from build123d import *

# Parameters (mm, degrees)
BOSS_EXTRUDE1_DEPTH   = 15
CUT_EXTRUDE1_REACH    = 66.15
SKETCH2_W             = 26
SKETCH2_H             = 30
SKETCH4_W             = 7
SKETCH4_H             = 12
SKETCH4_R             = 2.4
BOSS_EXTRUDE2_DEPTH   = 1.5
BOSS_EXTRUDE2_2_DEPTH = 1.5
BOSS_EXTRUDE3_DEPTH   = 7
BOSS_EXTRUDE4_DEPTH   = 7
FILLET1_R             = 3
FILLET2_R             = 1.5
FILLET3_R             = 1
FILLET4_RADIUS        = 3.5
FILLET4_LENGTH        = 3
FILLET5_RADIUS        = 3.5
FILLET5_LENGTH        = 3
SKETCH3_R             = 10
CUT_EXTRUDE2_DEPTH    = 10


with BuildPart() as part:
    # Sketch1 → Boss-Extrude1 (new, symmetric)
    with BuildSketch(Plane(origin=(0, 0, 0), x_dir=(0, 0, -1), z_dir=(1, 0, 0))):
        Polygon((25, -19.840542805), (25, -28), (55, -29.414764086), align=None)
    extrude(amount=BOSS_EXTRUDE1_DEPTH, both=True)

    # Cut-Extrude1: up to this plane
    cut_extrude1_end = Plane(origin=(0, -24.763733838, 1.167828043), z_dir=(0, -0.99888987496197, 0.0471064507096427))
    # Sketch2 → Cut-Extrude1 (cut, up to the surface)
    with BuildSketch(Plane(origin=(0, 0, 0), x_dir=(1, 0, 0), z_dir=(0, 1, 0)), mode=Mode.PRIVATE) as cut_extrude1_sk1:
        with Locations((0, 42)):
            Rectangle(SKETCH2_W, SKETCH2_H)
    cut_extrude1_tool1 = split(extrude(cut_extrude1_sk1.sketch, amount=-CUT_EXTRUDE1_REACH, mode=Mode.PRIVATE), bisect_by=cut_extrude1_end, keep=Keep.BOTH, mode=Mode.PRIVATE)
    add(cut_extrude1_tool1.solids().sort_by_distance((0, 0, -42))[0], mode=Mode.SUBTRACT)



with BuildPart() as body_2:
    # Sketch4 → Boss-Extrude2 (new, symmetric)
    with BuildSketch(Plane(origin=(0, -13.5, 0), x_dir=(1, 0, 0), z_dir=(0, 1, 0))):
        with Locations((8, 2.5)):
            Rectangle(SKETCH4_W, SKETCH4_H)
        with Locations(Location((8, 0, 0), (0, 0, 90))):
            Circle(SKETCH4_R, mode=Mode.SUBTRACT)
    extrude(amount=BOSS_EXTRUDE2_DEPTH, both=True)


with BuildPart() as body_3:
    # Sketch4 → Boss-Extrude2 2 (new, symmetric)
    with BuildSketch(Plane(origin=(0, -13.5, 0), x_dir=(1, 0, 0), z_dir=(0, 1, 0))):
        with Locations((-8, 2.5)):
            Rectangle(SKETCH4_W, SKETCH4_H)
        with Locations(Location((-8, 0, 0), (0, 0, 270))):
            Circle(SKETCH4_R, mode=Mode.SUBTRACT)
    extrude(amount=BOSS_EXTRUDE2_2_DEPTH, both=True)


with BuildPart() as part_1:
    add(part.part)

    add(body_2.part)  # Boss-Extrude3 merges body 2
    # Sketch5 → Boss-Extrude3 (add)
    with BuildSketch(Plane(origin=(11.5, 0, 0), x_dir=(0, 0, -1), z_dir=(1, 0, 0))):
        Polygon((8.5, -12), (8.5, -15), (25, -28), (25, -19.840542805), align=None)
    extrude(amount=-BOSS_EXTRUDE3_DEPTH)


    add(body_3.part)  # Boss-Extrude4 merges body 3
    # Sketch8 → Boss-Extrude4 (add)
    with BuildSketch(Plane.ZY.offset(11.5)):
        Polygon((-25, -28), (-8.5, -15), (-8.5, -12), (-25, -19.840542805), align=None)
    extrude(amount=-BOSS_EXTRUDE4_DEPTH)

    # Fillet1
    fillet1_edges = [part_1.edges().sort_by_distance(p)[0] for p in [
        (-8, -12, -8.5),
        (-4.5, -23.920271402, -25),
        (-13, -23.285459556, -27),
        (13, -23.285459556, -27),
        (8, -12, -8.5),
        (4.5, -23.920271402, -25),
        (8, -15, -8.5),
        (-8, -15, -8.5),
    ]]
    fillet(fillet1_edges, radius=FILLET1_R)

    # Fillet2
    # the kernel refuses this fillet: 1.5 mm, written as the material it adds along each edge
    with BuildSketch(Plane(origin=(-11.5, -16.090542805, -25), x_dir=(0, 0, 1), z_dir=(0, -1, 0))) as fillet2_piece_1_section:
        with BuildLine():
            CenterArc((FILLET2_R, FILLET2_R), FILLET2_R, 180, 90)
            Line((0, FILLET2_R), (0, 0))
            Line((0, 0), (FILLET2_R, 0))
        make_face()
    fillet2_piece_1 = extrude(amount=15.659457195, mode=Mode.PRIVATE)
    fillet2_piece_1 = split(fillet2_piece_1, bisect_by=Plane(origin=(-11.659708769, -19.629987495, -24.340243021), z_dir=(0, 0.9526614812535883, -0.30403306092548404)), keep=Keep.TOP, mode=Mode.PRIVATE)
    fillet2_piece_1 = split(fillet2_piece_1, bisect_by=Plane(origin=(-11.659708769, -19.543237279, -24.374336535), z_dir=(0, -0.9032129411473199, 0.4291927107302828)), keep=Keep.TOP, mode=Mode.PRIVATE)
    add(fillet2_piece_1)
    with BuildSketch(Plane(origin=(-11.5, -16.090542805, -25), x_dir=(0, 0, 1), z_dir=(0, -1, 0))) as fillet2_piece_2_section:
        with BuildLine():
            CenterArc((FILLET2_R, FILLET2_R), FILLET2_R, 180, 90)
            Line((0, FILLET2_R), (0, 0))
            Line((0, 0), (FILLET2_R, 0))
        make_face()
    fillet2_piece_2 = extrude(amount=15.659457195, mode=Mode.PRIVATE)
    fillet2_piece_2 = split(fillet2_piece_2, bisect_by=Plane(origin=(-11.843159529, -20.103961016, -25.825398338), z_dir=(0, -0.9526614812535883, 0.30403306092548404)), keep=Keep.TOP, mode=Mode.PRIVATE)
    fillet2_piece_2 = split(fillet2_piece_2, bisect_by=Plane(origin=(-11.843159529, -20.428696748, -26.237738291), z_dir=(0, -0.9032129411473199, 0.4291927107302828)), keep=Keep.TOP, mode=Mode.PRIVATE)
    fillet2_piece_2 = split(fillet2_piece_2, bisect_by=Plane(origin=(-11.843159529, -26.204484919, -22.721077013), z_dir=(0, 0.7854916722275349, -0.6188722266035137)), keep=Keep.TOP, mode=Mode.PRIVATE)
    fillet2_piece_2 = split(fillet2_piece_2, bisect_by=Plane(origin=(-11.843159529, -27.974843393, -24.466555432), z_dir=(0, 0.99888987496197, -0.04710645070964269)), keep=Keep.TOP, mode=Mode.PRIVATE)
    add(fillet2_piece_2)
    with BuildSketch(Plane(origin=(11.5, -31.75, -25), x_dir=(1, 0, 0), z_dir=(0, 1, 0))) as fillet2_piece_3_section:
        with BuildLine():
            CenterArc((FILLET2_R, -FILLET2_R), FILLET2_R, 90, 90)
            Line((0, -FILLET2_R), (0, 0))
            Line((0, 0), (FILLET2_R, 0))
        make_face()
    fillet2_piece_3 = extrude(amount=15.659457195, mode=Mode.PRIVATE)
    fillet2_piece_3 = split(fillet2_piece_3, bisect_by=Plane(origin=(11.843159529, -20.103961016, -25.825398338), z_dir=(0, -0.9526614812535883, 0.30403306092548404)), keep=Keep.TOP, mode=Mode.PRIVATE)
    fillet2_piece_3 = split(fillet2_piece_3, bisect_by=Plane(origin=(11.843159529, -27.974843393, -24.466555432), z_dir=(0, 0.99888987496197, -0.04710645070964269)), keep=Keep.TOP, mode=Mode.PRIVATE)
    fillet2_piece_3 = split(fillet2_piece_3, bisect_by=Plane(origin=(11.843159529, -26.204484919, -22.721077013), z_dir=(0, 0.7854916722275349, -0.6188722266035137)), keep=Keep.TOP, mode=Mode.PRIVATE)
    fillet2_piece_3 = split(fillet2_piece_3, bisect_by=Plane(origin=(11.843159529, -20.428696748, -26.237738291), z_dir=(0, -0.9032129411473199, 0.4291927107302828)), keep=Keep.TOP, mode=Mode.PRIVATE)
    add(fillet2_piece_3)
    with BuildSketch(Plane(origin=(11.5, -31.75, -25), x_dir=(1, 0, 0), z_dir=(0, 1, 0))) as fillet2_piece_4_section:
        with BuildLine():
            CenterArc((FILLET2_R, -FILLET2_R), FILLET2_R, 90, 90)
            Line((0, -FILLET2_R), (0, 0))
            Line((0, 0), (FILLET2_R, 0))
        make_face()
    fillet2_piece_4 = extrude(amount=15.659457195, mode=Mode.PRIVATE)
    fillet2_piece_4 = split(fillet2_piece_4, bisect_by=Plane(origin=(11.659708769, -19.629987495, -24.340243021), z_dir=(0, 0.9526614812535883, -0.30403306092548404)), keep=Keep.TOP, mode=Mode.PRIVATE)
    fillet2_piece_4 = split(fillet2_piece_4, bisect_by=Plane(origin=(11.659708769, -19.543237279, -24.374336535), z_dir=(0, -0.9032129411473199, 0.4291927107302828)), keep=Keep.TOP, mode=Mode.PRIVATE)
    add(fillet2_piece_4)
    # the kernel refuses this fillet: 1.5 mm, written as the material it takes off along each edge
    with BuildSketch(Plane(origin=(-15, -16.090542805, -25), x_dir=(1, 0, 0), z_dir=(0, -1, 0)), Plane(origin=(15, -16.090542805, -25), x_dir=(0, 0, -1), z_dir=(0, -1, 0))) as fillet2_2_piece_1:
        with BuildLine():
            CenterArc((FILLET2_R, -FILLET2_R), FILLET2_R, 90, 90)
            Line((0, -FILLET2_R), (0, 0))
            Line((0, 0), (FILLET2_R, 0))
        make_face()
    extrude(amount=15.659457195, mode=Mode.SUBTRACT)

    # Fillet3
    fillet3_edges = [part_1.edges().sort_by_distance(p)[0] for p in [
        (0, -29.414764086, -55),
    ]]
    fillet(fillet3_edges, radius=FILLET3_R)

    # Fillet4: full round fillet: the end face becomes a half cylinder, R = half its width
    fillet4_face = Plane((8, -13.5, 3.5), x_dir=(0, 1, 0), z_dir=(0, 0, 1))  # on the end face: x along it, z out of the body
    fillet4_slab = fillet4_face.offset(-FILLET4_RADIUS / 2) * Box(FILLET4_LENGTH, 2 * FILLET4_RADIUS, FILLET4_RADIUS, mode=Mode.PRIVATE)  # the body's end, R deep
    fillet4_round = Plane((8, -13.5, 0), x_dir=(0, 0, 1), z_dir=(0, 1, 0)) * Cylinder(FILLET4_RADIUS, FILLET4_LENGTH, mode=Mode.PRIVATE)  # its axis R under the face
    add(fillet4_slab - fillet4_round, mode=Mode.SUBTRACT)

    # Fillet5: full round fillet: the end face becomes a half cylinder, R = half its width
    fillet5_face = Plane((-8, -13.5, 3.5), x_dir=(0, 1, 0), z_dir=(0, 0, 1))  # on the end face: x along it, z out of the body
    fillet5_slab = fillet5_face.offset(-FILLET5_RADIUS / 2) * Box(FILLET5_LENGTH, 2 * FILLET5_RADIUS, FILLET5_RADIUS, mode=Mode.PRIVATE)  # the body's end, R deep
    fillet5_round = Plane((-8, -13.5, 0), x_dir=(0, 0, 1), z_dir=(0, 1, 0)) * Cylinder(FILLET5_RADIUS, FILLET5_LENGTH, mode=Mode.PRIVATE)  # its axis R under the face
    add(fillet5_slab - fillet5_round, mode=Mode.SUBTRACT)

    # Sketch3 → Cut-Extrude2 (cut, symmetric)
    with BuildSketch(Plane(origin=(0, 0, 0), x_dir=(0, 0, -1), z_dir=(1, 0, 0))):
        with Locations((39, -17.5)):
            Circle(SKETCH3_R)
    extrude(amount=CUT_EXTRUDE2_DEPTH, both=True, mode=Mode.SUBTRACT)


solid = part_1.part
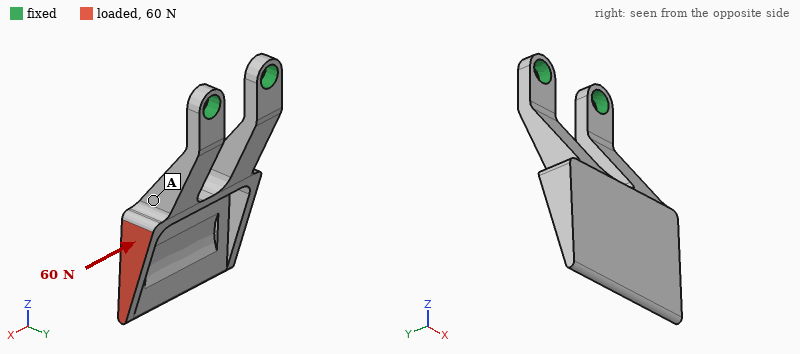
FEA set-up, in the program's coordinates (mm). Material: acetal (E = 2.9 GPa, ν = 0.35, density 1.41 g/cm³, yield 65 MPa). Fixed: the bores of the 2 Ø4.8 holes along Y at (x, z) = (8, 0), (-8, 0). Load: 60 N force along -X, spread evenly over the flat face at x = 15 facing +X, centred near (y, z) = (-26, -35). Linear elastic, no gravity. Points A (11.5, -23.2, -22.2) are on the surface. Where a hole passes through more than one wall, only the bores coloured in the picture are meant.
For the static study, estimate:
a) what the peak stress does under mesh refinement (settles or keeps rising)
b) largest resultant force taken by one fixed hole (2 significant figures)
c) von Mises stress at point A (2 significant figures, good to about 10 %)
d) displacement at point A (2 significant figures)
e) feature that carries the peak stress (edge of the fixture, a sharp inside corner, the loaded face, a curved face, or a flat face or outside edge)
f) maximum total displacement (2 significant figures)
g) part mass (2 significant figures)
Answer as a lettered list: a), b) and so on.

a) keeps rising
b) 87 N
c) 3.0 MPa
d) 0.31 mm
e) edge of the fixture
f) 0.71 mm
g) 5.1 g
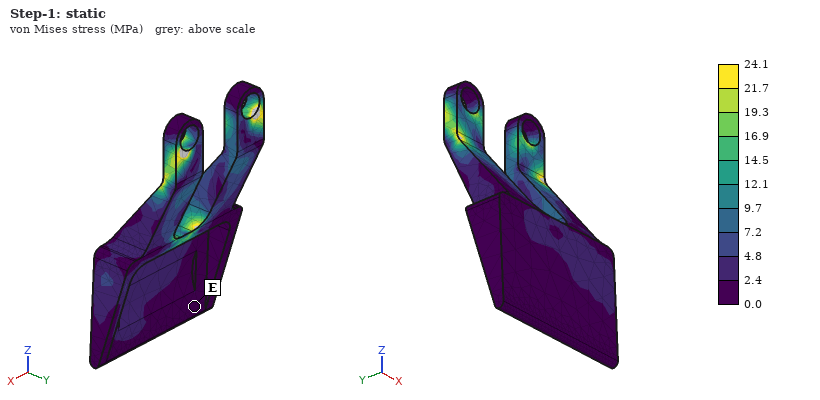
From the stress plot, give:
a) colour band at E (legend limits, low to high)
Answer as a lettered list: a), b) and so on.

a) 0.0 to 2.4 MPa
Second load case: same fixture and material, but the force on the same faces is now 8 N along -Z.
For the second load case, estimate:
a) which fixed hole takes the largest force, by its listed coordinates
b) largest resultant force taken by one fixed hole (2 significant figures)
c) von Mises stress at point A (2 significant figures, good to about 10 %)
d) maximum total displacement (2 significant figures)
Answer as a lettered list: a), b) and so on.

a) (8, 0)
b) 9.2 N
c) 1.0 MPa
d) 0.67 mm
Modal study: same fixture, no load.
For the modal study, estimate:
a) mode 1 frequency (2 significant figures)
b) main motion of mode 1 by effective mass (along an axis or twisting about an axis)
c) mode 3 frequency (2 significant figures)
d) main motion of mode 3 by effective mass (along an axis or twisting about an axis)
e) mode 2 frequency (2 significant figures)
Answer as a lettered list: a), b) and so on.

a) 260 Hz
b) along Y
c) 1000 Hz
d) along X
e) 820 Hz
